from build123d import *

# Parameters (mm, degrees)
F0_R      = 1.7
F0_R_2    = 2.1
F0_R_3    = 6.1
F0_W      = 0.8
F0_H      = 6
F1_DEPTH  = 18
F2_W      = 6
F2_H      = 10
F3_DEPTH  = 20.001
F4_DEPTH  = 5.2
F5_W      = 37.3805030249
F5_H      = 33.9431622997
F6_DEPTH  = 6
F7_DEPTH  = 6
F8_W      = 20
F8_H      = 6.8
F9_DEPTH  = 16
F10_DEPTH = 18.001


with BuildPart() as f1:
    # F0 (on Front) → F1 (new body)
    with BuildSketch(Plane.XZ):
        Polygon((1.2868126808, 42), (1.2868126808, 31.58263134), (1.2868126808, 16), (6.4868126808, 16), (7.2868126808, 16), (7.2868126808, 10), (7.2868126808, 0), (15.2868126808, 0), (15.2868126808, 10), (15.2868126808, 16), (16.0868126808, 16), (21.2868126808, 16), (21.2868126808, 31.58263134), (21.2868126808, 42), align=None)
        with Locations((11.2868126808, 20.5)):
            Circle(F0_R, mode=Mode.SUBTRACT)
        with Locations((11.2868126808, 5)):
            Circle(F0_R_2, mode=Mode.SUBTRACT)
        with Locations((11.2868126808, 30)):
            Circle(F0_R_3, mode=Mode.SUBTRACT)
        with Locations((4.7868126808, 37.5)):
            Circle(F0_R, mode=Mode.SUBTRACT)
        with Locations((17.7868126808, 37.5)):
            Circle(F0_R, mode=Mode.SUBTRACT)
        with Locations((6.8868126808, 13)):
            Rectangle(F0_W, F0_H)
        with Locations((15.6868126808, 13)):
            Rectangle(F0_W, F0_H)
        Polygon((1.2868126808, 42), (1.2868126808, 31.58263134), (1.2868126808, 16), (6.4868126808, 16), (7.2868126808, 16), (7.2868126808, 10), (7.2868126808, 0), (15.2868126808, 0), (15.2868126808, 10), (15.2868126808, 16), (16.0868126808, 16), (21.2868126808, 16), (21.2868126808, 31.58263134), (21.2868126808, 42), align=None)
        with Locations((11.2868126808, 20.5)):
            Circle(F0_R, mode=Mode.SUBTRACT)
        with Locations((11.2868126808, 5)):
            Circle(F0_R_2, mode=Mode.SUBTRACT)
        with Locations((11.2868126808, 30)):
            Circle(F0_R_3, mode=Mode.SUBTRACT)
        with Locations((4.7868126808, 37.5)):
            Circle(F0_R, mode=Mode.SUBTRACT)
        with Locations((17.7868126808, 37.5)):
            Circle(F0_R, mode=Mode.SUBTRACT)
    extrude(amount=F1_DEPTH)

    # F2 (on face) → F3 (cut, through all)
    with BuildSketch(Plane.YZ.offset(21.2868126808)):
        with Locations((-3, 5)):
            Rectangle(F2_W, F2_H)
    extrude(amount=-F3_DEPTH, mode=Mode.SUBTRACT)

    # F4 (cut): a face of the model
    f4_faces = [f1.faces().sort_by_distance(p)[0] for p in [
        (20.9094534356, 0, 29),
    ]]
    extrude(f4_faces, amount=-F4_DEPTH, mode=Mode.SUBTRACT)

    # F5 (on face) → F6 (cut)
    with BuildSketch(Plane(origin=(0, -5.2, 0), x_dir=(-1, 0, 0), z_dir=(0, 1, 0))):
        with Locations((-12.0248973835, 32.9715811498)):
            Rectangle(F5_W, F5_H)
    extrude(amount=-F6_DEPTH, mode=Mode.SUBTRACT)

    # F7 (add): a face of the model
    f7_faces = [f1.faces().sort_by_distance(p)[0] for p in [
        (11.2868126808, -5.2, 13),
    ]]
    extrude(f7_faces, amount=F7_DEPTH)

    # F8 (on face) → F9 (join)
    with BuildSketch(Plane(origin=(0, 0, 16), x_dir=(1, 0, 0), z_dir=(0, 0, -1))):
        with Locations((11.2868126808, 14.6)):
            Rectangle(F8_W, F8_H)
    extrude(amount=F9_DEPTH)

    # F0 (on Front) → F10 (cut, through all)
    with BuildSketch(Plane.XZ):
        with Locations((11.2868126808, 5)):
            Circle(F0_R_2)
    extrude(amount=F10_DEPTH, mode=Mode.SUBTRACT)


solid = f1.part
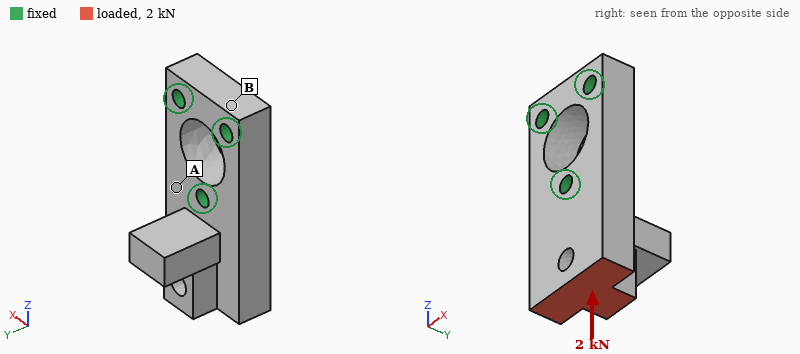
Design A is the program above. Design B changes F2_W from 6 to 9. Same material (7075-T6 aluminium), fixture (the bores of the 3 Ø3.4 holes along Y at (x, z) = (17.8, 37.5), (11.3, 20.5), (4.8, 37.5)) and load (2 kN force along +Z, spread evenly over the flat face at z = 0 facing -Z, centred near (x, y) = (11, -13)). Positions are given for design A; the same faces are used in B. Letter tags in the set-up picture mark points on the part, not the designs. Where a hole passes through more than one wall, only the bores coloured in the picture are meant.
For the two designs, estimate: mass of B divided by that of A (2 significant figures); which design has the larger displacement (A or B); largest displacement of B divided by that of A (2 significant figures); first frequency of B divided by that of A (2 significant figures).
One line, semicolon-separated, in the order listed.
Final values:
0.98; A; 0.71; 1.0
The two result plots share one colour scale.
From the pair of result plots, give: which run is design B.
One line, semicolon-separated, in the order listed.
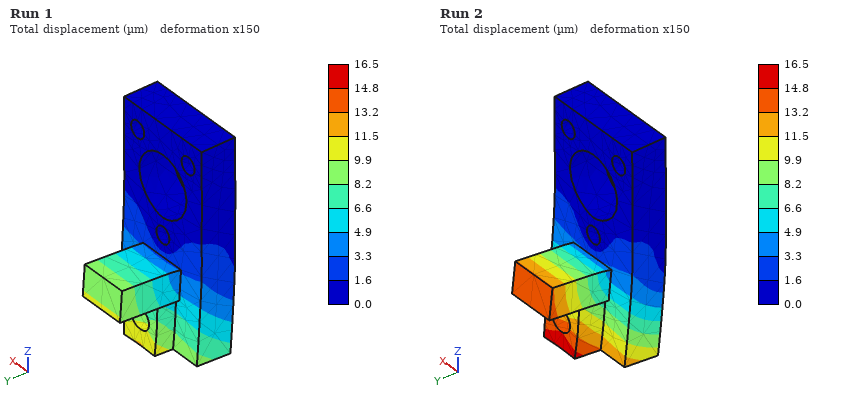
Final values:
Run 1
